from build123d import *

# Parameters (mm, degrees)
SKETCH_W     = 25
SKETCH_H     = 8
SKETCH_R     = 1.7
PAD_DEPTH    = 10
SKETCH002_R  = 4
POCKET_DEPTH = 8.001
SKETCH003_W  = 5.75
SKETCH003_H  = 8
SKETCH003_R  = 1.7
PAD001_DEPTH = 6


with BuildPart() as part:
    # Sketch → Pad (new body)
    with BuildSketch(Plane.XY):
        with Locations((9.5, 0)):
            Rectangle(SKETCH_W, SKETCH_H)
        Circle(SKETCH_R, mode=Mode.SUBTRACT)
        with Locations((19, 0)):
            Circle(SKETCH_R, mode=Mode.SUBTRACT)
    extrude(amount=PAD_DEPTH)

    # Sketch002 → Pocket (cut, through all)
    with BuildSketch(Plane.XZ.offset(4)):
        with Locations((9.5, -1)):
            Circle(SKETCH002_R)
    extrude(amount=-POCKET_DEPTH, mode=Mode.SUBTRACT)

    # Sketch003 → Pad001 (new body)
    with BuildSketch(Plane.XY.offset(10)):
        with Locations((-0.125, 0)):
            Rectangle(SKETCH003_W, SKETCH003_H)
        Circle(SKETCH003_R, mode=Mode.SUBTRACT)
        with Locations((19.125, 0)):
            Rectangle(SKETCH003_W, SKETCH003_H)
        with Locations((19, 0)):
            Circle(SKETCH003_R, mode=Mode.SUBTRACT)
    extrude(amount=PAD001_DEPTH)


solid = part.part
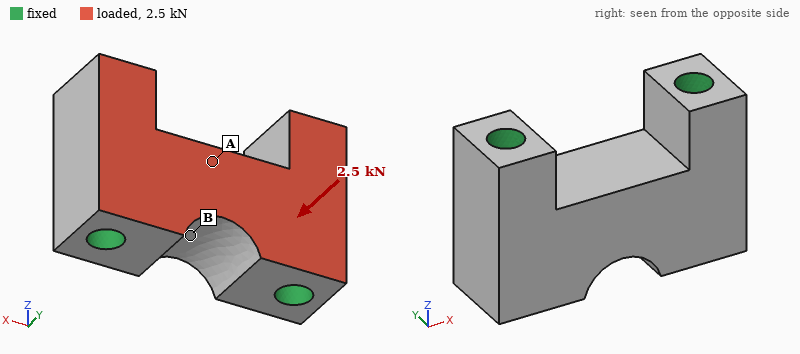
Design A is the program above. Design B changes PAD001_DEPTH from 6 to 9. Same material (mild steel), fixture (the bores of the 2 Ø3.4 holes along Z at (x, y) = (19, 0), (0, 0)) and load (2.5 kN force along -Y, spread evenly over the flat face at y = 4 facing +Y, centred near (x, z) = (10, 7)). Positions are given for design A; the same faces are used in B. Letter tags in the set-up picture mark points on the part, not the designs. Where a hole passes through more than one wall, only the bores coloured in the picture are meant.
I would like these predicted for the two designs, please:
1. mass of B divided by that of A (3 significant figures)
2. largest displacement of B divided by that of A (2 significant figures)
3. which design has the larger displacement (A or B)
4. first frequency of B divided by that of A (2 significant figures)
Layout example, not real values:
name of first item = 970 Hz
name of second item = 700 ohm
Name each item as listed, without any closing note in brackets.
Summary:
mass of B divided by that of A = 1.10
largest displacement of B divided by that of A = 0.90
which design has the larger displacement = A
first frequency of B divided by that of A = 1.0
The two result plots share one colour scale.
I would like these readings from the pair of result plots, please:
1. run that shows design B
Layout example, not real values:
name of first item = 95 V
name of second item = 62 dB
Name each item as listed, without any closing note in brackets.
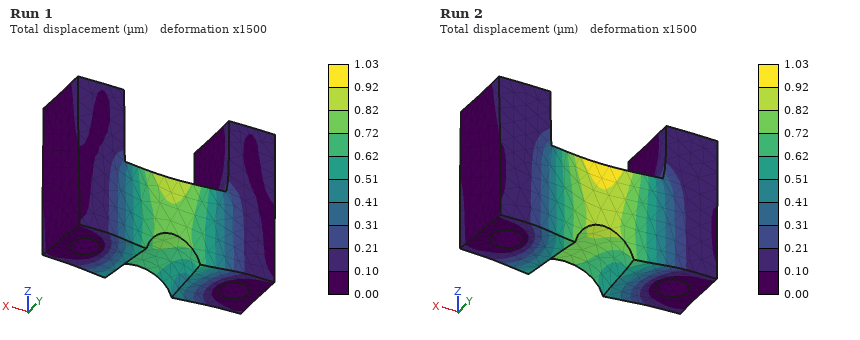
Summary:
run that shows design B = Run 1
